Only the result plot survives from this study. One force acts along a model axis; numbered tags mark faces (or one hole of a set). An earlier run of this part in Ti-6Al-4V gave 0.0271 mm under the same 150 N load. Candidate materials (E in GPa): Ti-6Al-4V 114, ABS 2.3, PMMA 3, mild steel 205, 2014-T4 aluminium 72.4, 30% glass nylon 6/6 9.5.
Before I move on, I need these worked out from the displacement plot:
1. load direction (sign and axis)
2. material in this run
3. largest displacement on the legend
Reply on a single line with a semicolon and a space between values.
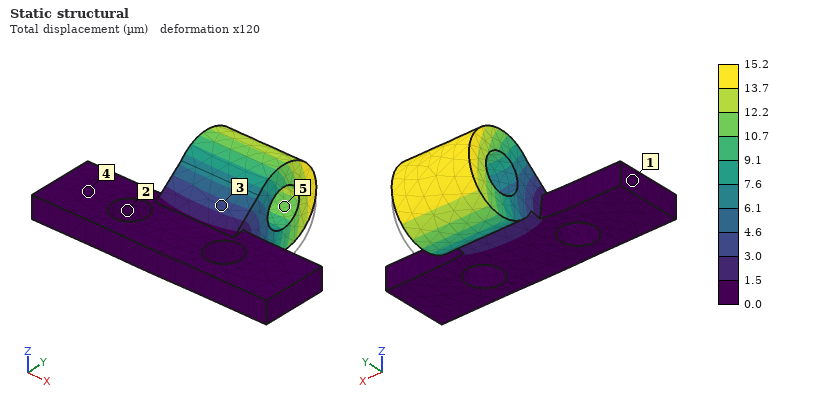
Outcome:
+Z; mild steel; 15.2 µm
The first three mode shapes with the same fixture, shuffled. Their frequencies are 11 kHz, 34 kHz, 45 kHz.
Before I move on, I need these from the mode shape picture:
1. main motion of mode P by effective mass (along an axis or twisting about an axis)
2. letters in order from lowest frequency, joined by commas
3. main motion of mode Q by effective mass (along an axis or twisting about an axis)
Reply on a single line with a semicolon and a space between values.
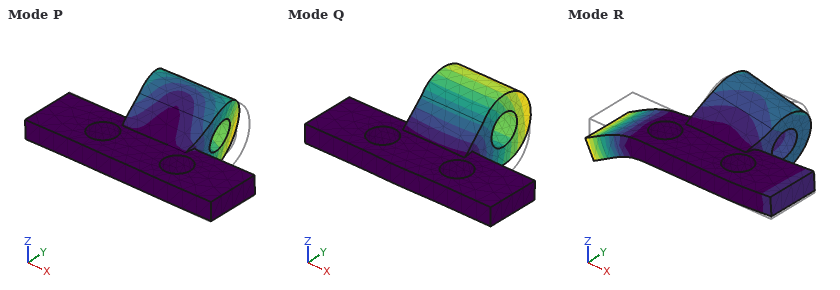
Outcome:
along X; Q, P, R; along Z
